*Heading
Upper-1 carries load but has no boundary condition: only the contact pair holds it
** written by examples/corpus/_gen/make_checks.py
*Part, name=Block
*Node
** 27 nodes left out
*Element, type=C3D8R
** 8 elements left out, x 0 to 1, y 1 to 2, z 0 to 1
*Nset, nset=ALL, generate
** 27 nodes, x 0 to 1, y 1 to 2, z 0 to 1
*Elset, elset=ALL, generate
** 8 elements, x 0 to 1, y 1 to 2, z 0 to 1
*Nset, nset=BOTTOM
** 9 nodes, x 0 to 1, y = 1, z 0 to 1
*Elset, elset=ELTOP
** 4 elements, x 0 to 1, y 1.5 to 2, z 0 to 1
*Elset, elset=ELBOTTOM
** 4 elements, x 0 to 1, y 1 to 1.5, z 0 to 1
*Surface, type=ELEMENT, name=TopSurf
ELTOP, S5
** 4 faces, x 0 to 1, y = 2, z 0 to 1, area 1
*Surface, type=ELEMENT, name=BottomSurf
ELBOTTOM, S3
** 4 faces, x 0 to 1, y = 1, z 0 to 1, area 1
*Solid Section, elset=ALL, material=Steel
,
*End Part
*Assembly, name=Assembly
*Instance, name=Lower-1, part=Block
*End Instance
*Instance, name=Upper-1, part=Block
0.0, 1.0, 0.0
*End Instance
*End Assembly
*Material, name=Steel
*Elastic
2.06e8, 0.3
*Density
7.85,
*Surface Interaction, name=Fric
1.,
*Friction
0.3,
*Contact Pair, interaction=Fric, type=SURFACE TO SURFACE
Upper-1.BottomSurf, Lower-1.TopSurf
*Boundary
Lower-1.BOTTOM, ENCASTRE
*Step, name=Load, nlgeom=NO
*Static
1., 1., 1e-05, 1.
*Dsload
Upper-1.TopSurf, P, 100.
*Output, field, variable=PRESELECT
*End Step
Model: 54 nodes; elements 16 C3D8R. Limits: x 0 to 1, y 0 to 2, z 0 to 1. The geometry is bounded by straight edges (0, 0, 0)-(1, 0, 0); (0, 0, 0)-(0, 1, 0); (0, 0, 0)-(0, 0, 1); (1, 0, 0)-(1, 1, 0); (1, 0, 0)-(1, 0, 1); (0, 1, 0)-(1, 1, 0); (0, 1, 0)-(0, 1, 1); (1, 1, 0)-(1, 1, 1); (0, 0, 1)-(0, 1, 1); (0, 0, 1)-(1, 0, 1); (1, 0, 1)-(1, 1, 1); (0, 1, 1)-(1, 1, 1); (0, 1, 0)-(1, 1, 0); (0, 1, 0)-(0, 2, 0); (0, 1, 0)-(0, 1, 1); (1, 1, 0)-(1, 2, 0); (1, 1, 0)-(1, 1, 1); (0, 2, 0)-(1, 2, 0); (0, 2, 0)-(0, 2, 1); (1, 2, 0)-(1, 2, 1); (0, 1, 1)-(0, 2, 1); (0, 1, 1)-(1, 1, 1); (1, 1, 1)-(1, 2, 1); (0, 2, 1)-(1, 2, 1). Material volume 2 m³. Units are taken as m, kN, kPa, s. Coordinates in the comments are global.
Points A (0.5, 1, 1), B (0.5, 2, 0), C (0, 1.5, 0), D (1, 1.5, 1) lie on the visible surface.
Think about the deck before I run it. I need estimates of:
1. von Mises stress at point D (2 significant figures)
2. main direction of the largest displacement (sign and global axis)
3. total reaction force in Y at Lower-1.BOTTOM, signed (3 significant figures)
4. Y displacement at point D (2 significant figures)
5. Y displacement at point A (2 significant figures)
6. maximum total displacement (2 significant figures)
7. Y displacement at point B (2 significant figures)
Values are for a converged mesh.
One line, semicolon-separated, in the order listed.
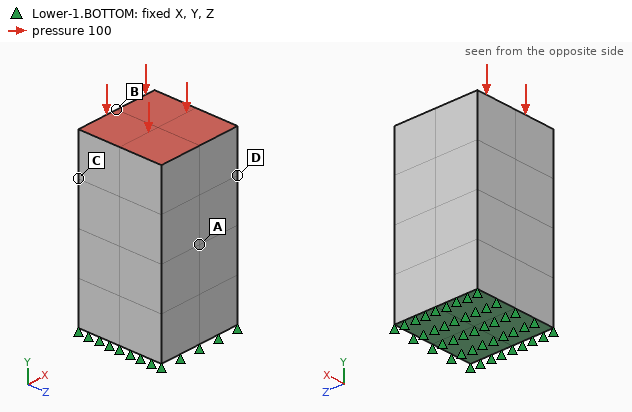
100 kPa; -Y; 100 kN; -7.2e-07 m; -4.8e-07 m; 9.7e-07 m; -9.6e-07 m
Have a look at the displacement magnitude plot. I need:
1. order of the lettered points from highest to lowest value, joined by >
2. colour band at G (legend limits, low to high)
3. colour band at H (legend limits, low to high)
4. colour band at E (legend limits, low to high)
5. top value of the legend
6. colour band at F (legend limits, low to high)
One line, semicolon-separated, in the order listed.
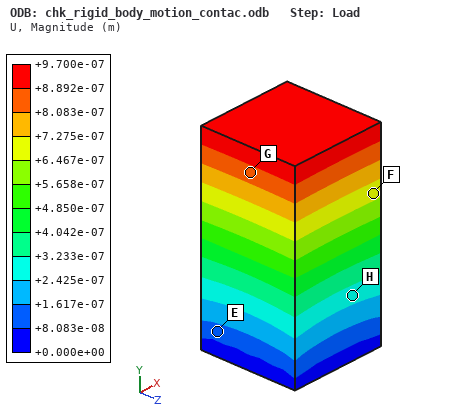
G > F > H > E; +8.083e-07 to +8.892e-07 m; +2.425e-07 to +3.233e-07 m; +8.083e-08 to +1.617e-07 m; +9.700e-07 m; +6.467e-07 to +7.275e-07 m
